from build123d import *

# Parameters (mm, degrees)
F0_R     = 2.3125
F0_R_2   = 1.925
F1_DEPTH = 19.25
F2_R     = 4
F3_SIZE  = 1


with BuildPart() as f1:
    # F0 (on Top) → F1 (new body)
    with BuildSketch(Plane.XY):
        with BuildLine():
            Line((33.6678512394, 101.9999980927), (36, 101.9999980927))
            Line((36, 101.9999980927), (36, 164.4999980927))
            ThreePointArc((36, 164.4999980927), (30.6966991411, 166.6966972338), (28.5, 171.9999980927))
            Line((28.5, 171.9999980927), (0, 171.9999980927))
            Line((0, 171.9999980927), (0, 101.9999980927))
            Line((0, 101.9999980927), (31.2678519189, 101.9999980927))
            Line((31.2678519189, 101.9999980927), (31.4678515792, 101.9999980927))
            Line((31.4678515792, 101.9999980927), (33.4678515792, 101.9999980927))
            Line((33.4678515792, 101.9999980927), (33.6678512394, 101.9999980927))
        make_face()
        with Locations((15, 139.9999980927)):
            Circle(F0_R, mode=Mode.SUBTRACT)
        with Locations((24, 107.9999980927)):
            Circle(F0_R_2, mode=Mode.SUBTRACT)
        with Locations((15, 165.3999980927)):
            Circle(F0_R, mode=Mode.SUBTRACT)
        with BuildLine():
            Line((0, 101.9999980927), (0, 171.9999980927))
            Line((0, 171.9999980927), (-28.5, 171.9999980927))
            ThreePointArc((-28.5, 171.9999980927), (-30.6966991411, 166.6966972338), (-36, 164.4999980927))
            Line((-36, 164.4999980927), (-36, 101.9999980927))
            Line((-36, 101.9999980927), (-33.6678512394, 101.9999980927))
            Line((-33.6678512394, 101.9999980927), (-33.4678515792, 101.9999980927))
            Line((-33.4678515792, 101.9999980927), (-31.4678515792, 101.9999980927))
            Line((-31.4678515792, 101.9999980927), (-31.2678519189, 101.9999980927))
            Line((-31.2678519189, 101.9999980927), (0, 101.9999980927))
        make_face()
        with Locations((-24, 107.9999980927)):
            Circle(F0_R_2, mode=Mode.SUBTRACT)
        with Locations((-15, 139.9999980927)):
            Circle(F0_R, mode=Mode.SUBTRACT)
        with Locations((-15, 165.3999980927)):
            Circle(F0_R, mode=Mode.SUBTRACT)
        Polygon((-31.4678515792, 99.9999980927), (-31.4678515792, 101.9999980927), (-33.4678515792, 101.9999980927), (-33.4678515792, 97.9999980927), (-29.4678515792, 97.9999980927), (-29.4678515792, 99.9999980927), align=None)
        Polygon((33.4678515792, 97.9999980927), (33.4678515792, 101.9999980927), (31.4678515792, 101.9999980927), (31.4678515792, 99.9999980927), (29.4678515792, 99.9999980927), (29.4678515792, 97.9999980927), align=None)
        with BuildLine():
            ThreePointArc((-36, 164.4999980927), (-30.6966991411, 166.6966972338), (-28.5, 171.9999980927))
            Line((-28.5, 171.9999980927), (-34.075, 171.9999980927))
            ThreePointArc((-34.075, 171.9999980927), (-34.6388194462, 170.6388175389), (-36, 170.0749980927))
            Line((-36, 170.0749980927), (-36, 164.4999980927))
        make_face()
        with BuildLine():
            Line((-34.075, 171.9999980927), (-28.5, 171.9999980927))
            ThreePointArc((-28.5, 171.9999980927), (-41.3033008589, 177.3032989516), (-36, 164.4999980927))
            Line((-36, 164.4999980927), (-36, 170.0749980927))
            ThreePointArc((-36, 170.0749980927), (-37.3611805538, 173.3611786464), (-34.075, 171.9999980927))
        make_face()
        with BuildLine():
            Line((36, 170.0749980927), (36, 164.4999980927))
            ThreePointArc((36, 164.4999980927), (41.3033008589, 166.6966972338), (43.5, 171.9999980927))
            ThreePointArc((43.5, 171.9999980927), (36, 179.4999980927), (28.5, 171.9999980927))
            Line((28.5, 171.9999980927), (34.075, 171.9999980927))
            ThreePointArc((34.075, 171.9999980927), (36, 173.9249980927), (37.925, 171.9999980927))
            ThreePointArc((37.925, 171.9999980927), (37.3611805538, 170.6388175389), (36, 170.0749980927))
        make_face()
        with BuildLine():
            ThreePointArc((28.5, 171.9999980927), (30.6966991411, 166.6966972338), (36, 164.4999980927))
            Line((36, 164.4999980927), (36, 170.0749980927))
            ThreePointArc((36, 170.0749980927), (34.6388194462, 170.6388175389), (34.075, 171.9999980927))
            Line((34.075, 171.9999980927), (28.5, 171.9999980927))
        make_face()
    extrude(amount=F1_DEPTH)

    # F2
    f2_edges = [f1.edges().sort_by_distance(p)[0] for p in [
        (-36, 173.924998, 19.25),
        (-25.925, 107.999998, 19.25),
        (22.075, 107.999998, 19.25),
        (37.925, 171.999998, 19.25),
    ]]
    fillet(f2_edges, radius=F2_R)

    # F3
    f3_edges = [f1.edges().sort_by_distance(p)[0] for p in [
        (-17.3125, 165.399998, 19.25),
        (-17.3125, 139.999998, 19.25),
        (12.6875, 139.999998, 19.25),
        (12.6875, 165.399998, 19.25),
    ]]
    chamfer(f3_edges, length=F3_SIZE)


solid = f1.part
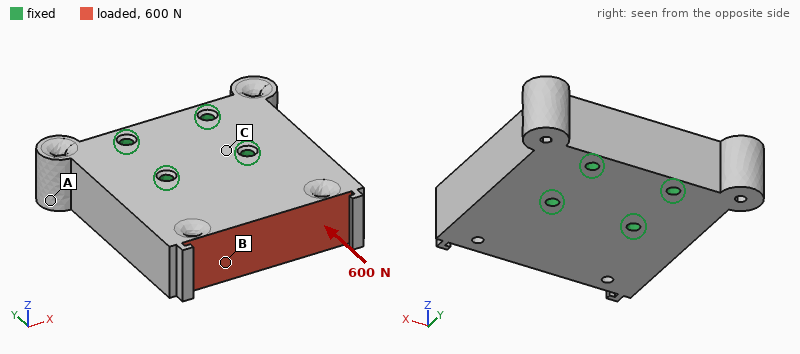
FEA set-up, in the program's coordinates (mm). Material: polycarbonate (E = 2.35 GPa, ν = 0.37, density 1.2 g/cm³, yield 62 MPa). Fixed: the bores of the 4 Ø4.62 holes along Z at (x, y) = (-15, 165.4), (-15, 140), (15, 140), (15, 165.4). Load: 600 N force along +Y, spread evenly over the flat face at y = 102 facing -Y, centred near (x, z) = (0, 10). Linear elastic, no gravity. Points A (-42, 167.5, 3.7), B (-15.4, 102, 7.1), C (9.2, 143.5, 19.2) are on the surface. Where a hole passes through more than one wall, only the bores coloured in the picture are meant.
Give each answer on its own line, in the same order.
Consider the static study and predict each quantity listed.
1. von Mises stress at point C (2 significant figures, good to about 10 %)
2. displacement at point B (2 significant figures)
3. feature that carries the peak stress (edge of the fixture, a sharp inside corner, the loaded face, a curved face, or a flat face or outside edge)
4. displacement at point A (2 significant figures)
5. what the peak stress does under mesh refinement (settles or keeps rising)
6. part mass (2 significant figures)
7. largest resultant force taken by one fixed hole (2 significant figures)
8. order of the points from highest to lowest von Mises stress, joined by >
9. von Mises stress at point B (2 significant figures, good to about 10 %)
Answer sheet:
0.31 MPa
9.4 µm
edge of the fixture
3.1 µm
keeps rising
120 g
240 N
B > C > A
0.52 MPa
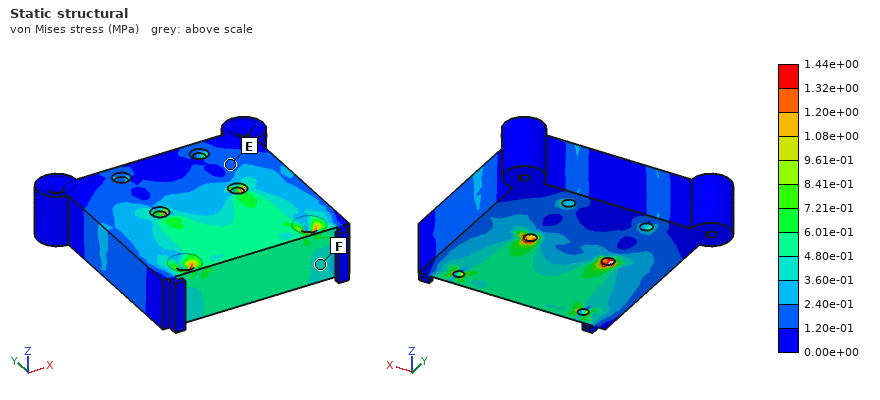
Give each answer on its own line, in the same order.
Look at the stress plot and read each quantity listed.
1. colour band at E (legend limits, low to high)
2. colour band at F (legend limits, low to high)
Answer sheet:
1.20e-01 to 2.40e-01 MPa
3.60e-01 to 4.80e-01 MPa
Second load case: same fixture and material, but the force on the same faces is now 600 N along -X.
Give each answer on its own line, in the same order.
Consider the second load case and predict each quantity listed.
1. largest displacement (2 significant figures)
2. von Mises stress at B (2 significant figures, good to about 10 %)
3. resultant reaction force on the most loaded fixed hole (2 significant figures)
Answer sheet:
58 µm
1.0 MPa
560 N
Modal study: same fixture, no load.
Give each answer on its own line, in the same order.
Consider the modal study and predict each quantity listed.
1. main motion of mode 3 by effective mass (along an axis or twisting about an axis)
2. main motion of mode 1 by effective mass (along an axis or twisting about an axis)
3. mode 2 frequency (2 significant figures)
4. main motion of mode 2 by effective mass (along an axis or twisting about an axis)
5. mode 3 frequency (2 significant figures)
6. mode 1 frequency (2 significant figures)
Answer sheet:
along X
along Z
2800 Hz
twisting about Y
3400 Hz
2100 Hz
